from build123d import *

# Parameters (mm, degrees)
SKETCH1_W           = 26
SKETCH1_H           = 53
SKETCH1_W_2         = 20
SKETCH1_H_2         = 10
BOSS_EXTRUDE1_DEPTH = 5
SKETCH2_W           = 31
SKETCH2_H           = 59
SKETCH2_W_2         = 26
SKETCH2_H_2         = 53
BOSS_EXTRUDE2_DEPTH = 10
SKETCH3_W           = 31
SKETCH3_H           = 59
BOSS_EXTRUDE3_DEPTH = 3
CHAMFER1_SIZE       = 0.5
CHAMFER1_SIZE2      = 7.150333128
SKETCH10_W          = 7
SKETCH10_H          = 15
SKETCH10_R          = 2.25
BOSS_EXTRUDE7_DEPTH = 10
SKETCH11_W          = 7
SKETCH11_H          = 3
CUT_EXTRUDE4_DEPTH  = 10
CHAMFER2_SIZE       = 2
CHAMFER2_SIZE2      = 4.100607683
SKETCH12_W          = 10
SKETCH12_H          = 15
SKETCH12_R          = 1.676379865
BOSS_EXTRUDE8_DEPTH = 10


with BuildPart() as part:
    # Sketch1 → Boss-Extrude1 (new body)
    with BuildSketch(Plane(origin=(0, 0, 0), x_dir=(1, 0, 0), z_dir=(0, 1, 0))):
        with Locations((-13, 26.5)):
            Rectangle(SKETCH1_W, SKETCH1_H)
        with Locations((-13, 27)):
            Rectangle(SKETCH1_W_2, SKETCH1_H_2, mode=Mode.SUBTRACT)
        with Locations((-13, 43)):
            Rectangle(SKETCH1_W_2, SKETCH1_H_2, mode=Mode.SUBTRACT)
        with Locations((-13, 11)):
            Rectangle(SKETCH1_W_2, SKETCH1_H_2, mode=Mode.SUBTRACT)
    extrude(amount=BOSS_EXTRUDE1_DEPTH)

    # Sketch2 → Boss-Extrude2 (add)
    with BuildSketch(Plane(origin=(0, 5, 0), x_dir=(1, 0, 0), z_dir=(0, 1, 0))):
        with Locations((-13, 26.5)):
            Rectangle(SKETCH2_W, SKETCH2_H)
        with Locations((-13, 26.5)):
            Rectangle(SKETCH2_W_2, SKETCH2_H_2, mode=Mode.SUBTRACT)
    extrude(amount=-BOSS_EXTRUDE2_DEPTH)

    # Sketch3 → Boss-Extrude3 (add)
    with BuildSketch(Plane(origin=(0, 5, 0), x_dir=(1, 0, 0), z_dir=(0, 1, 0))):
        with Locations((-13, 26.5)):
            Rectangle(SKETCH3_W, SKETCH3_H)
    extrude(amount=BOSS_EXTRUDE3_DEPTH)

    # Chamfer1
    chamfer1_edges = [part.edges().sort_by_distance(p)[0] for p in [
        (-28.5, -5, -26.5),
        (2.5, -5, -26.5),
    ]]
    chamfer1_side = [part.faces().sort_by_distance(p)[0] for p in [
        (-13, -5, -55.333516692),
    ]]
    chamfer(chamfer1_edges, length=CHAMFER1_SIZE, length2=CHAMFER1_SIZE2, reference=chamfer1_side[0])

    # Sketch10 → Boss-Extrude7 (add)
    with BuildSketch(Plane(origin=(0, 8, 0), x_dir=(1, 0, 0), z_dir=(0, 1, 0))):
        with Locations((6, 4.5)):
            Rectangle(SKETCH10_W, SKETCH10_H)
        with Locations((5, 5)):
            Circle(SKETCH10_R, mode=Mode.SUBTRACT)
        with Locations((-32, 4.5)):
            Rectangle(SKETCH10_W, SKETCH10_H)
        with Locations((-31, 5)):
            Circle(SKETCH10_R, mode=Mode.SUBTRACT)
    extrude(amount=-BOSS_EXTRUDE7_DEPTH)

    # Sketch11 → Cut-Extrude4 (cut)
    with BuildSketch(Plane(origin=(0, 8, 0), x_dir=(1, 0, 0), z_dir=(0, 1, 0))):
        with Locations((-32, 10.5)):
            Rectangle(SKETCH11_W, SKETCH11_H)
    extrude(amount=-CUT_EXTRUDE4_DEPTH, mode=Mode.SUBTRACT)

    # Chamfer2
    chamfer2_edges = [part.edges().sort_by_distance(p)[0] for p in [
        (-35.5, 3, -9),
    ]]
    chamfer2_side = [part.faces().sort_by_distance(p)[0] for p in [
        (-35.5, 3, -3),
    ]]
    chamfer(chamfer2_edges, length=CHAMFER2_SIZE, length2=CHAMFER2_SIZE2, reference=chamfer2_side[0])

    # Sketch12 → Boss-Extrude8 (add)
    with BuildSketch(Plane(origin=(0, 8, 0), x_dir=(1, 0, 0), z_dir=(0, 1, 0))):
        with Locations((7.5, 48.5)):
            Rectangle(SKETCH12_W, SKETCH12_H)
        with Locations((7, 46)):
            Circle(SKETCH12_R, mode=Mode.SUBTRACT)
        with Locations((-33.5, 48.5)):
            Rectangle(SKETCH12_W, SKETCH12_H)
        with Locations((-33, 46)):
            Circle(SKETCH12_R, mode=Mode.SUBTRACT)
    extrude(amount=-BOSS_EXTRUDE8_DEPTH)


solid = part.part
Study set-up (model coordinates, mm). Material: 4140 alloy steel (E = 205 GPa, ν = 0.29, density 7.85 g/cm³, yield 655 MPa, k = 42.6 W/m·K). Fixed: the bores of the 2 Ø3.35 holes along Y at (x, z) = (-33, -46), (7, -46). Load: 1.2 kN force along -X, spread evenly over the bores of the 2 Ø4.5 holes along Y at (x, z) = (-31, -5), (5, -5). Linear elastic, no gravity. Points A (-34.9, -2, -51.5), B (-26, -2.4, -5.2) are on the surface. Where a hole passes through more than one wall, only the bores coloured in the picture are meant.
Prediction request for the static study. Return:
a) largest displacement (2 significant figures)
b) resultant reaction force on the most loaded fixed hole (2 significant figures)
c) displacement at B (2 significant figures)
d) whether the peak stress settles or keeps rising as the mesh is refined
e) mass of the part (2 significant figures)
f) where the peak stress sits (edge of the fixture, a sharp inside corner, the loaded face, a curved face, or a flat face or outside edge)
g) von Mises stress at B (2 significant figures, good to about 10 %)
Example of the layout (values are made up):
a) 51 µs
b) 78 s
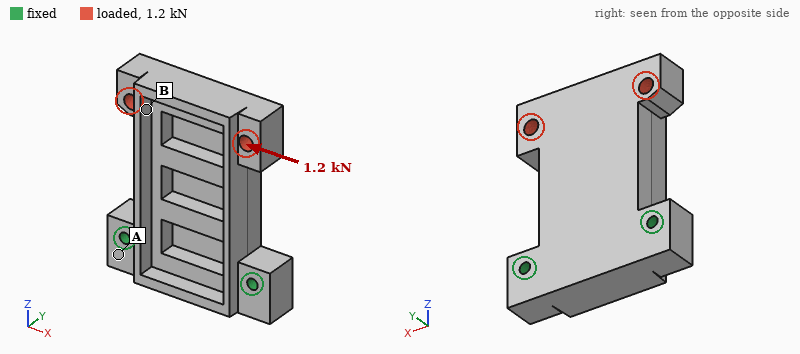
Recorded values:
a) 35 µm
b) 1.5 kN
c) 25 µm
d) keeps rising
e) 140 g
f) edge of the fixture
g) 20 MPa
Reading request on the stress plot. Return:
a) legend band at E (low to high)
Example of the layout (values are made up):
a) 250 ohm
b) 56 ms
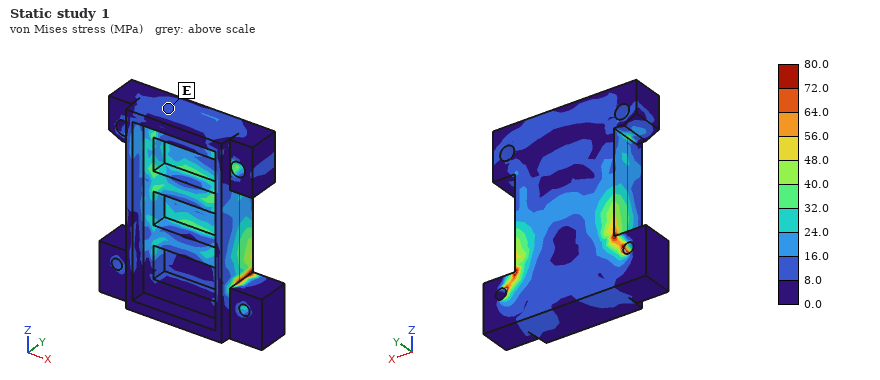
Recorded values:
a) 8.0 to 16.0 MPa
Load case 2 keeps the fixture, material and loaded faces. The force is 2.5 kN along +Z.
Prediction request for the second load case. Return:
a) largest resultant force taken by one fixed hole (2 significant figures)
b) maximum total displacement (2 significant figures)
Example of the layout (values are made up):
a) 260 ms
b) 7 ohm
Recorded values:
a) 1.3 kN
b) 17 µm
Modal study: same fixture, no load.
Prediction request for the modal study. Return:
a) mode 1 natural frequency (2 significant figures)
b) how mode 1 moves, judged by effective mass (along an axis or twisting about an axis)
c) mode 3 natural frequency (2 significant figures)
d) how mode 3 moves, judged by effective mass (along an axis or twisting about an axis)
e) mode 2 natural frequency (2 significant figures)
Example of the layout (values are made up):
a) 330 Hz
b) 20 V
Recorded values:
a) 1900 Hz
b) along Y
c) 6300 Hz
d) along X
e) 3700 Hz
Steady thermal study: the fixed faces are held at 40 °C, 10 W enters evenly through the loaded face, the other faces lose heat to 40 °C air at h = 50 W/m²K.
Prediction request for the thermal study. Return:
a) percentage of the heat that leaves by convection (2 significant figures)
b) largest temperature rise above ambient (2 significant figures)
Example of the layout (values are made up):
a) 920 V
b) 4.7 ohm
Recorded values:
a) 65 %
b) 39 K
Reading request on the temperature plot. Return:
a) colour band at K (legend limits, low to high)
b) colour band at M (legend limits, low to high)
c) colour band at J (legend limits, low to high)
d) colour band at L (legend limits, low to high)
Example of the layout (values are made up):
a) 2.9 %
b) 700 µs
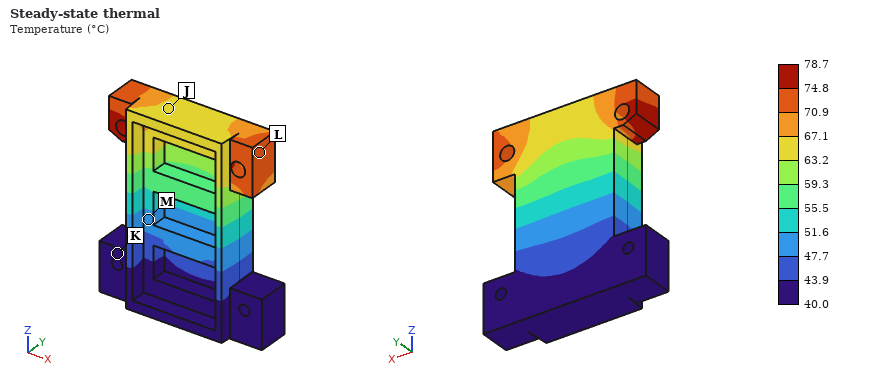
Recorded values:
a) 40.0 to 43.9 °C
b) 47.7 to 51.6 °C
c) 63.2 to 67.1 °C
d) 70.9 to 74.8 °C
